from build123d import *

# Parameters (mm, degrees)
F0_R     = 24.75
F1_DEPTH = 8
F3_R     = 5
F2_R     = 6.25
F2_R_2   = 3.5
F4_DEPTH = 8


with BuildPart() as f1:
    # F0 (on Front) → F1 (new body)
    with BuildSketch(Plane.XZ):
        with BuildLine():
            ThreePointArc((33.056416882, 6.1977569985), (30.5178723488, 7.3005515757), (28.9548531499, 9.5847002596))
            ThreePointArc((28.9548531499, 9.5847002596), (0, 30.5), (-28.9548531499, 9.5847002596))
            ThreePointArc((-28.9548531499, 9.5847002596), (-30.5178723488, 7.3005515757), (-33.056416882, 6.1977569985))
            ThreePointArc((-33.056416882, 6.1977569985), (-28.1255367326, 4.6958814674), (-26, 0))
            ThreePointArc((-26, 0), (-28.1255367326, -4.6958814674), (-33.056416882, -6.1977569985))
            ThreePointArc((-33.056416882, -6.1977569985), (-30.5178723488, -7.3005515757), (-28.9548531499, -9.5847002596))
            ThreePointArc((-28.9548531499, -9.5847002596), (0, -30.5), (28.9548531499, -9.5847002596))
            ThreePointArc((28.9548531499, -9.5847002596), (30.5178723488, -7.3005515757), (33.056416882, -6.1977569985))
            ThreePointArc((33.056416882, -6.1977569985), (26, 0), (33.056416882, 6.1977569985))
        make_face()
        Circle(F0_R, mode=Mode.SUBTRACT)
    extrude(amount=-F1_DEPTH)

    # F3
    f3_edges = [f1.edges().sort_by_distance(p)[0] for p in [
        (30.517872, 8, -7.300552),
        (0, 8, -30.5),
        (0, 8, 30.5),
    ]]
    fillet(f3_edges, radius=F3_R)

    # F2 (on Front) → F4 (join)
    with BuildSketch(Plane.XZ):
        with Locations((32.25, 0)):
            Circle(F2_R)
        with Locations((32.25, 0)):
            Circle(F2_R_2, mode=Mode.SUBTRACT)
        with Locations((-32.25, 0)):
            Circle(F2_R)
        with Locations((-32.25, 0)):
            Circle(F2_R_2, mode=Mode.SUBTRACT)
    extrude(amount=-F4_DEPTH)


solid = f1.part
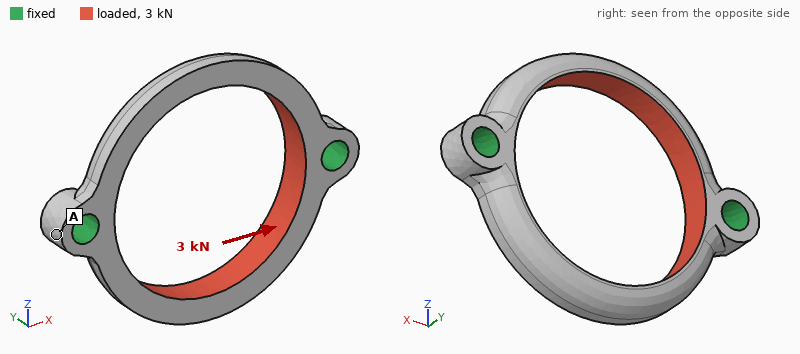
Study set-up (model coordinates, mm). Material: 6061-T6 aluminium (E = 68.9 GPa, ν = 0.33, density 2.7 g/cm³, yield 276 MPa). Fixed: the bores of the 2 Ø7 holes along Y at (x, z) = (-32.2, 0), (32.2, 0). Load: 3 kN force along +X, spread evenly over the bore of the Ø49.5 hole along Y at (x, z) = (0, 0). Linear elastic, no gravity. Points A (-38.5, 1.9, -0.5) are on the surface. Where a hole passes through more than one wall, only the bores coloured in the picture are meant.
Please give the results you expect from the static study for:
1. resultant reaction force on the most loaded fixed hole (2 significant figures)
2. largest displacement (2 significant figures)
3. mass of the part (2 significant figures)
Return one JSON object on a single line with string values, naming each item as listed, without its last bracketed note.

{"resultant reaction force on the most loaded fixed hole": "1.5 kN", "largest displacement": "54 µm", "mass of the part": "21 g"}
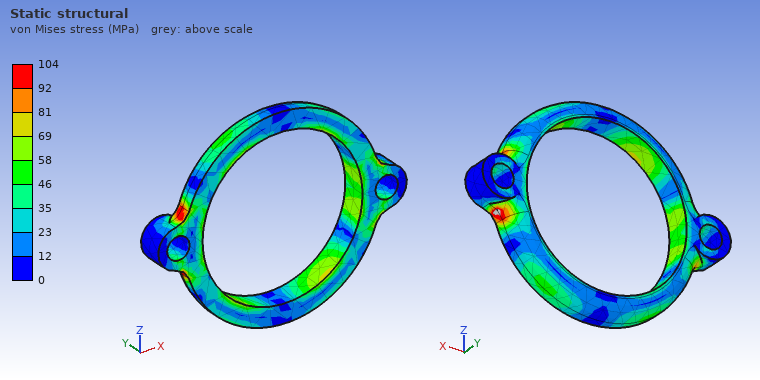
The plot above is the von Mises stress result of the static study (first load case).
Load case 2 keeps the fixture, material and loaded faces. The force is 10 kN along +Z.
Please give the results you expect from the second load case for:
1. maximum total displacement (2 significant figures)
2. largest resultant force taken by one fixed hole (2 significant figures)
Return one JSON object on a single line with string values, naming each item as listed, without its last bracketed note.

{"maximum total displacement": "58 µm", "largest resultant force taken by one fixed hole": "5.0 kN"}
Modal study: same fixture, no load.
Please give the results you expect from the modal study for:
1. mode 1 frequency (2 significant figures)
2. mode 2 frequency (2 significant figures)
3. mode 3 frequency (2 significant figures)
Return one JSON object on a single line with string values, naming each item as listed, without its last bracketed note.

{"mode 1 frequency": "4500 Hz", "mode 2 frequency": "4700 Hz", "mode 3 frequency": "8600 Hz"}
